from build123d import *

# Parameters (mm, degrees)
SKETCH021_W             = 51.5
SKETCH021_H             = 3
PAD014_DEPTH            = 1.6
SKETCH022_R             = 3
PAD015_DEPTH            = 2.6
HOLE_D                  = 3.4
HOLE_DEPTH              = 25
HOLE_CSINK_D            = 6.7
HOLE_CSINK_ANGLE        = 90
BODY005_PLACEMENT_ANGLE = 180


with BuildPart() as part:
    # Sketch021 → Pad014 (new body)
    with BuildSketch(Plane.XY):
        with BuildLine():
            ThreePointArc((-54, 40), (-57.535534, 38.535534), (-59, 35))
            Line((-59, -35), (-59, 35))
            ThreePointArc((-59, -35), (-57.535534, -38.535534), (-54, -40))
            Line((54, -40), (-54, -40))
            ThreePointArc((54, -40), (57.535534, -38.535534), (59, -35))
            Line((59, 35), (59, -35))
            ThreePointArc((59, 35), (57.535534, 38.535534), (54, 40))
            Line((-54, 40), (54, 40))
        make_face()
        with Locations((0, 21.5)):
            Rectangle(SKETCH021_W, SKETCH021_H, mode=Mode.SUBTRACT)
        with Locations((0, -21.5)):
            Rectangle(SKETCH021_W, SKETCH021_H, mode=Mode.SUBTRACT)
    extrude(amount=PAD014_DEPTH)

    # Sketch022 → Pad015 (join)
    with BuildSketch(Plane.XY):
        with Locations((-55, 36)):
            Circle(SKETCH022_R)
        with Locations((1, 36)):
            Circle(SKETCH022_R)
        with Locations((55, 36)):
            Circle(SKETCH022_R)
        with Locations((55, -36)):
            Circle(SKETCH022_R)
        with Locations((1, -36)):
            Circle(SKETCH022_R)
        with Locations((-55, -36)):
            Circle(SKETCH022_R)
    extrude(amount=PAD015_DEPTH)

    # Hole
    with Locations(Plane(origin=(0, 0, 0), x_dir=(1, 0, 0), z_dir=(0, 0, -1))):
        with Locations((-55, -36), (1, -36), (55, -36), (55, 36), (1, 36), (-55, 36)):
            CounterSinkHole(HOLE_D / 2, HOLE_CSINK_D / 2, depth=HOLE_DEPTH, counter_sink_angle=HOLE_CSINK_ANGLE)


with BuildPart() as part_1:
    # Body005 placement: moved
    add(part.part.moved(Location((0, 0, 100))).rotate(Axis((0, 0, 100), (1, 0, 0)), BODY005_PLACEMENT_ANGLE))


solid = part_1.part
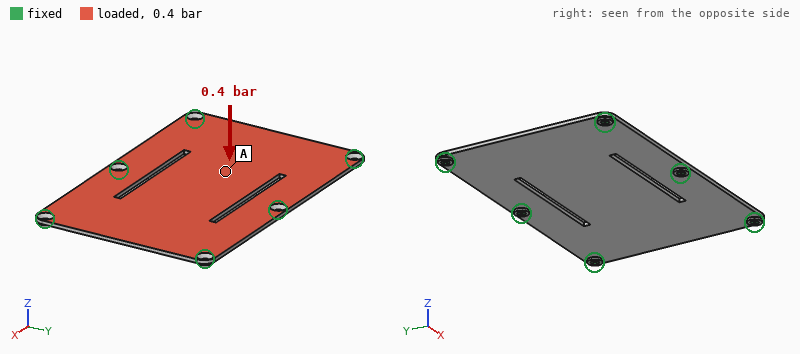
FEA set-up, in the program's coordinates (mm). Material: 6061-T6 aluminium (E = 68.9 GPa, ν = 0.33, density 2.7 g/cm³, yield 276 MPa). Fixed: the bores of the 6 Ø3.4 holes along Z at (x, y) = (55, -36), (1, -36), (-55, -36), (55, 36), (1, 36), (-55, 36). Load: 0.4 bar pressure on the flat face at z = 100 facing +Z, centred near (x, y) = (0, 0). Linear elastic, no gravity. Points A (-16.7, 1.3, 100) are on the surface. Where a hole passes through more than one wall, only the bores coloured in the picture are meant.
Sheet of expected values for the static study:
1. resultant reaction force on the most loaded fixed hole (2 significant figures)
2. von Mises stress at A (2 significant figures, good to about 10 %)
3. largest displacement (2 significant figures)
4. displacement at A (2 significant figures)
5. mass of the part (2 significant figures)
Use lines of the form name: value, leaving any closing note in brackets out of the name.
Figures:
resultant reaction force on the most loaded fixed hole: 160 N
von Mises stress at A: 23 MPa
largest displacement: 0.44 mm
displacement at A: 0.39 mm
mass of the part: 39 g
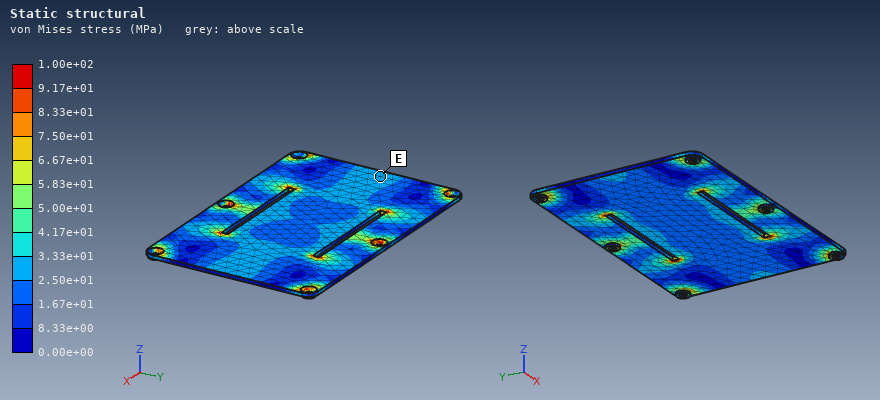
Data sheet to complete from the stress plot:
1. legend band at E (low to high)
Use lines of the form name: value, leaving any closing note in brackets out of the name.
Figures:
legend band at E: 2.50e+01 to 3.33e+01 MPa
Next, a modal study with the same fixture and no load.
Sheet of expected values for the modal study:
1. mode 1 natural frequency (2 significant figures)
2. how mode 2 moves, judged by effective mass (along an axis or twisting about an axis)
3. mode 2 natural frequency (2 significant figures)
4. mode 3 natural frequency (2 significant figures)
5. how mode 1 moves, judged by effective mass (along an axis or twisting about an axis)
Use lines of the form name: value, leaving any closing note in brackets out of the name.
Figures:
mode 1 natural frequency: 890 Hz
how mode 2 moves, judged by effective mass: twisting about Y
mode 2 natural frequency: 1400 Hz
mode 3 natural frequency: 1800 Hz
how mode 1 moves, judged by effective mass: along Z
